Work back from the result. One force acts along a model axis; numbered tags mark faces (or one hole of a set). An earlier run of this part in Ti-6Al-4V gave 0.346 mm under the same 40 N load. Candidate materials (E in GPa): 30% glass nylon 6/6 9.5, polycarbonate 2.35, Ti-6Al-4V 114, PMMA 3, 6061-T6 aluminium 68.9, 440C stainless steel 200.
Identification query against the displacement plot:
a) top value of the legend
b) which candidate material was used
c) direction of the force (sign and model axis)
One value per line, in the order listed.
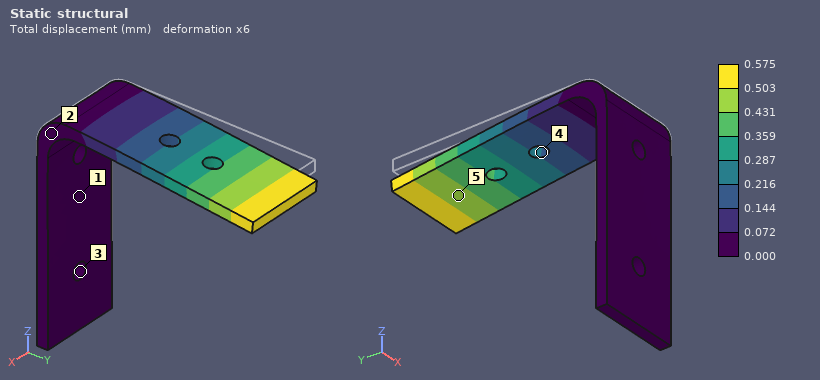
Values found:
0.575 mm
6061-T6 aluminium
-Z
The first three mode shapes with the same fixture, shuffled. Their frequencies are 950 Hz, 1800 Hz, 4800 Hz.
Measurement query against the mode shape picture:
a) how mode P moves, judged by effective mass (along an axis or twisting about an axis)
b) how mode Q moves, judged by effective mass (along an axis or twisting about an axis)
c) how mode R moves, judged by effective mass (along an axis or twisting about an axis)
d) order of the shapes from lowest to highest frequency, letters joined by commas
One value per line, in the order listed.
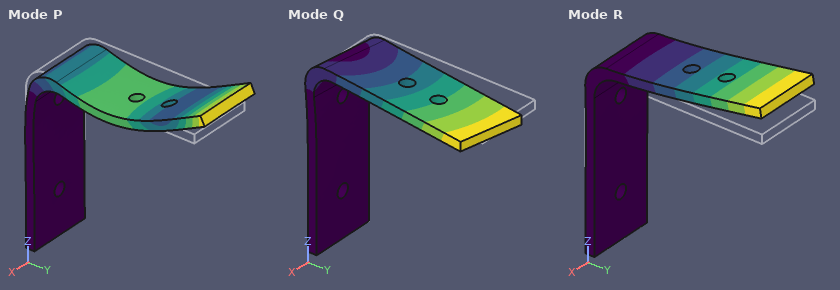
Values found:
along Y
along X
along Z
R, Q, P
